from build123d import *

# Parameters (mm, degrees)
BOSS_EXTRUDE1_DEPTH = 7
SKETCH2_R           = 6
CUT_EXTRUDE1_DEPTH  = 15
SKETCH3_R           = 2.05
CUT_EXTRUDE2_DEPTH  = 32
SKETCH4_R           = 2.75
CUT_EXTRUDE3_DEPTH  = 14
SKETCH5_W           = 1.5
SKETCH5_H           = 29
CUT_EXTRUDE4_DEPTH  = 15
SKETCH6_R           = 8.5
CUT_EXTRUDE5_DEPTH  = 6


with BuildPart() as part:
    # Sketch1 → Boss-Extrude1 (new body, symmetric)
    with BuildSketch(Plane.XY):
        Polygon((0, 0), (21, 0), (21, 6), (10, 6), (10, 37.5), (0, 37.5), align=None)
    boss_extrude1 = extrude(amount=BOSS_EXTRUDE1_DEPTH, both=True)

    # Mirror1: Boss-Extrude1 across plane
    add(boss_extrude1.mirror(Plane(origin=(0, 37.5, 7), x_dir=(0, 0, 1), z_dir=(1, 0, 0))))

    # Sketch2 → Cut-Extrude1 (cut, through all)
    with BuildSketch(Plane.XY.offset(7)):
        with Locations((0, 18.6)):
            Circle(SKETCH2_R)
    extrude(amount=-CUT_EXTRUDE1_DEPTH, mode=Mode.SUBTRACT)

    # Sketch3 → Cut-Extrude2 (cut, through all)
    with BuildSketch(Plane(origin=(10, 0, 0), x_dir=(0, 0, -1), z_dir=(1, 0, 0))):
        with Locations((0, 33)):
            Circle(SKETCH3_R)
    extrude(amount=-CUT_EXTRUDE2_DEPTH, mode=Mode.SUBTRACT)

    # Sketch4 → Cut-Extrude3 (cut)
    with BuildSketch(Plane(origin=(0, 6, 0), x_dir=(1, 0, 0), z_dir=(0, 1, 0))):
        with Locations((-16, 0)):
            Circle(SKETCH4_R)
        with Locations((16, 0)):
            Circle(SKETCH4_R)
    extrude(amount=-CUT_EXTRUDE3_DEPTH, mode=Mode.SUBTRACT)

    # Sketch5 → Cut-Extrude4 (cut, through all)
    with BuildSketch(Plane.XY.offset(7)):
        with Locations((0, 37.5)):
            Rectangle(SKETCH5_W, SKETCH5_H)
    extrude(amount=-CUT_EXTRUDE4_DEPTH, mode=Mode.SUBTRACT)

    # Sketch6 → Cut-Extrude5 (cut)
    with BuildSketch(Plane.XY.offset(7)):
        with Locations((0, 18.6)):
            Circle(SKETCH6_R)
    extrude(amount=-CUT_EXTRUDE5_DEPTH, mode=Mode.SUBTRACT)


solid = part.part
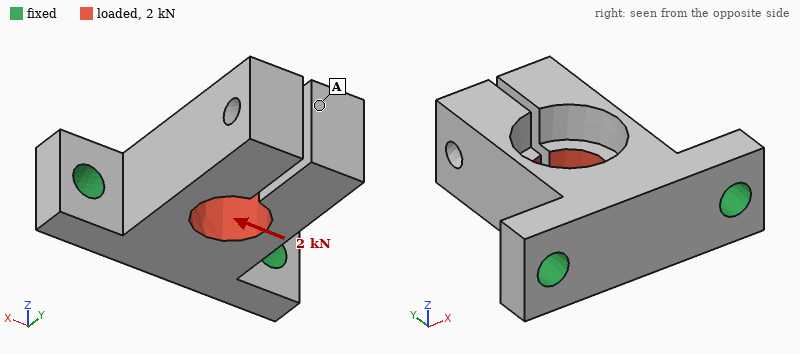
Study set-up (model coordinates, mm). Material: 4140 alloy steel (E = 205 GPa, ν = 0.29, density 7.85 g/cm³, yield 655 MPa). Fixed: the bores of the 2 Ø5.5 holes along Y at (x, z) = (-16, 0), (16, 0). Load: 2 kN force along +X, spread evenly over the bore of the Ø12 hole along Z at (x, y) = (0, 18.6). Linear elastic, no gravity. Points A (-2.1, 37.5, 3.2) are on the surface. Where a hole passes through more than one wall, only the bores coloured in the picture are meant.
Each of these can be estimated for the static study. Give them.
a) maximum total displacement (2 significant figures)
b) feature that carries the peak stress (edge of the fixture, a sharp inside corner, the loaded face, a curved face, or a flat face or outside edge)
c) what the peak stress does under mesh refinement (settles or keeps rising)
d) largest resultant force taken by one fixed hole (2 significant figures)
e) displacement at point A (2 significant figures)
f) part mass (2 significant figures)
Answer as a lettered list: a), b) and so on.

a) 54 µm
b) a sharp inside corner
c) keeps rising
d) 1.6 kN
e) 52 µm
f) 73 g
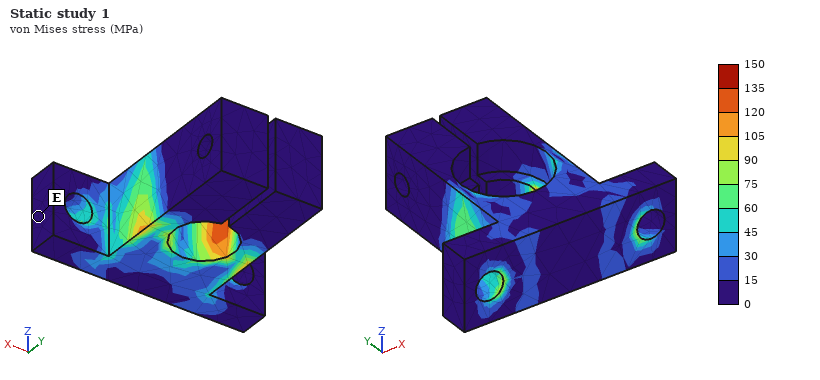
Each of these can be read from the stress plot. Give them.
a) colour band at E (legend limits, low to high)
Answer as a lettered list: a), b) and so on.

a) 0 to 15 MPa
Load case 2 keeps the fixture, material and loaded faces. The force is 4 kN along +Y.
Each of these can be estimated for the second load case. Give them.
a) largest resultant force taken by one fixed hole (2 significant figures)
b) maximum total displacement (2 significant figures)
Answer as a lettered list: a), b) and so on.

a) 2.2 kN
b) 72 µm
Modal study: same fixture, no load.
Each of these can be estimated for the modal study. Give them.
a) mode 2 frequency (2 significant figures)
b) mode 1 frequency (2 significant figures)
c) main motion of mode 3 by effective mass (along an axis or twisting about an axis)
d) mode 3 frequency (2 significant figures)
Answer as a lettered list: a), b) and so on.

a) 3300 Hz
b) 3300 Hz
c) along Z
d) 4100 Hz
